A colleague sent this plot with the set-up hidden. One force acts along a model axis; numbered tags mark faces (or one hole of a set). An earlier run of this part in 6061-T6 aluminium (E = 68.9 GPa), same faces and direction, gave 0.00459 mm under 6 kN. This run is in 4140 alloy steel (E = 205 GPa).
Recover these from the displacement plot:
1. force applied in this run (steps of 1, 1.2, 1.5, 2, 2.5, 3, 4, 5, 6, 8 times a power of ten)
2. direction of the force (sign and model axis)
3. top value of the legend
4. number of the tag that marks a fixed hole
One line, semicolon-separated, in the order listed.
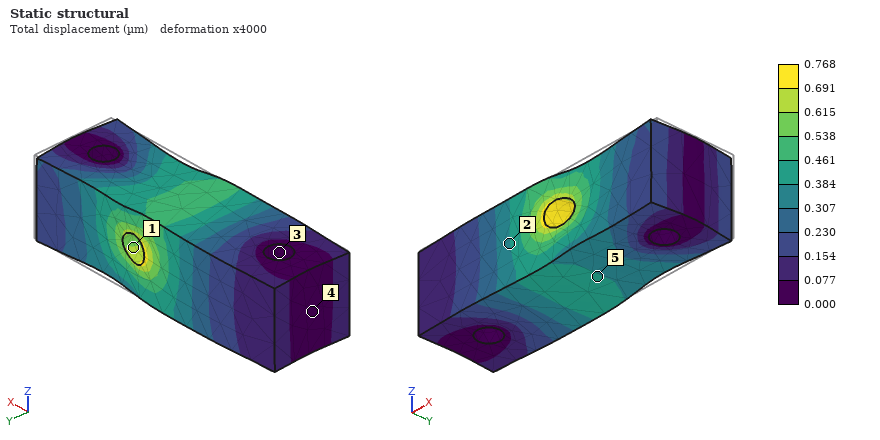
3 kN; -X; 0.768 µm; 3
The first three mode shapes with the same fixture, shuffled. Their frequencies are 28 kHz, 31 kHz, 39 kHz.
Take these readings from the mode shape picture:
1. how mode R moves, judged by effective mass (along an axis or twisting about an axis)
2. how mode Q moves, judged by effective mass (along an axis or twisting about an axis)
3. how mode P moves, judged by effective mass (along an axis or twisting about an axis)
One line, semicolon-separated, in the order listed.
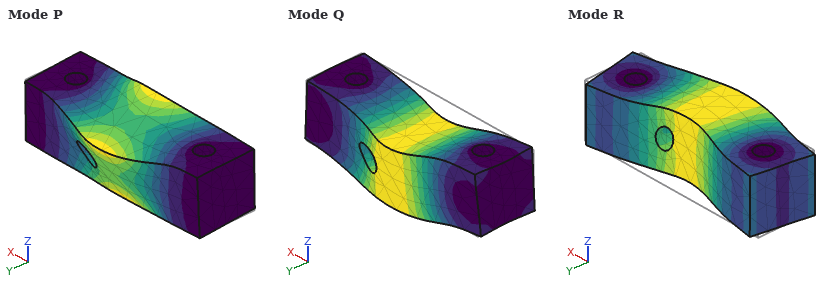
along Y; along Z; twisting about X
